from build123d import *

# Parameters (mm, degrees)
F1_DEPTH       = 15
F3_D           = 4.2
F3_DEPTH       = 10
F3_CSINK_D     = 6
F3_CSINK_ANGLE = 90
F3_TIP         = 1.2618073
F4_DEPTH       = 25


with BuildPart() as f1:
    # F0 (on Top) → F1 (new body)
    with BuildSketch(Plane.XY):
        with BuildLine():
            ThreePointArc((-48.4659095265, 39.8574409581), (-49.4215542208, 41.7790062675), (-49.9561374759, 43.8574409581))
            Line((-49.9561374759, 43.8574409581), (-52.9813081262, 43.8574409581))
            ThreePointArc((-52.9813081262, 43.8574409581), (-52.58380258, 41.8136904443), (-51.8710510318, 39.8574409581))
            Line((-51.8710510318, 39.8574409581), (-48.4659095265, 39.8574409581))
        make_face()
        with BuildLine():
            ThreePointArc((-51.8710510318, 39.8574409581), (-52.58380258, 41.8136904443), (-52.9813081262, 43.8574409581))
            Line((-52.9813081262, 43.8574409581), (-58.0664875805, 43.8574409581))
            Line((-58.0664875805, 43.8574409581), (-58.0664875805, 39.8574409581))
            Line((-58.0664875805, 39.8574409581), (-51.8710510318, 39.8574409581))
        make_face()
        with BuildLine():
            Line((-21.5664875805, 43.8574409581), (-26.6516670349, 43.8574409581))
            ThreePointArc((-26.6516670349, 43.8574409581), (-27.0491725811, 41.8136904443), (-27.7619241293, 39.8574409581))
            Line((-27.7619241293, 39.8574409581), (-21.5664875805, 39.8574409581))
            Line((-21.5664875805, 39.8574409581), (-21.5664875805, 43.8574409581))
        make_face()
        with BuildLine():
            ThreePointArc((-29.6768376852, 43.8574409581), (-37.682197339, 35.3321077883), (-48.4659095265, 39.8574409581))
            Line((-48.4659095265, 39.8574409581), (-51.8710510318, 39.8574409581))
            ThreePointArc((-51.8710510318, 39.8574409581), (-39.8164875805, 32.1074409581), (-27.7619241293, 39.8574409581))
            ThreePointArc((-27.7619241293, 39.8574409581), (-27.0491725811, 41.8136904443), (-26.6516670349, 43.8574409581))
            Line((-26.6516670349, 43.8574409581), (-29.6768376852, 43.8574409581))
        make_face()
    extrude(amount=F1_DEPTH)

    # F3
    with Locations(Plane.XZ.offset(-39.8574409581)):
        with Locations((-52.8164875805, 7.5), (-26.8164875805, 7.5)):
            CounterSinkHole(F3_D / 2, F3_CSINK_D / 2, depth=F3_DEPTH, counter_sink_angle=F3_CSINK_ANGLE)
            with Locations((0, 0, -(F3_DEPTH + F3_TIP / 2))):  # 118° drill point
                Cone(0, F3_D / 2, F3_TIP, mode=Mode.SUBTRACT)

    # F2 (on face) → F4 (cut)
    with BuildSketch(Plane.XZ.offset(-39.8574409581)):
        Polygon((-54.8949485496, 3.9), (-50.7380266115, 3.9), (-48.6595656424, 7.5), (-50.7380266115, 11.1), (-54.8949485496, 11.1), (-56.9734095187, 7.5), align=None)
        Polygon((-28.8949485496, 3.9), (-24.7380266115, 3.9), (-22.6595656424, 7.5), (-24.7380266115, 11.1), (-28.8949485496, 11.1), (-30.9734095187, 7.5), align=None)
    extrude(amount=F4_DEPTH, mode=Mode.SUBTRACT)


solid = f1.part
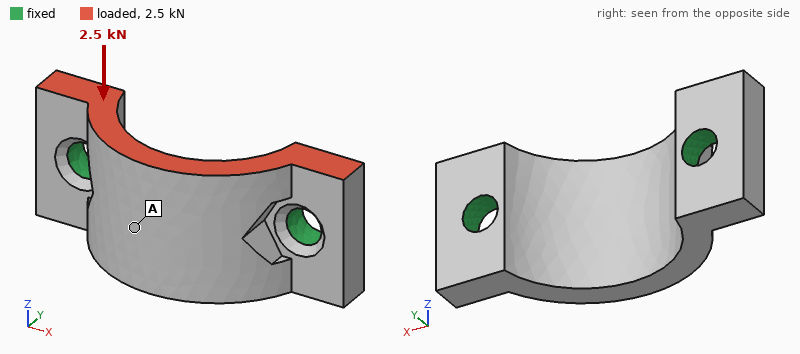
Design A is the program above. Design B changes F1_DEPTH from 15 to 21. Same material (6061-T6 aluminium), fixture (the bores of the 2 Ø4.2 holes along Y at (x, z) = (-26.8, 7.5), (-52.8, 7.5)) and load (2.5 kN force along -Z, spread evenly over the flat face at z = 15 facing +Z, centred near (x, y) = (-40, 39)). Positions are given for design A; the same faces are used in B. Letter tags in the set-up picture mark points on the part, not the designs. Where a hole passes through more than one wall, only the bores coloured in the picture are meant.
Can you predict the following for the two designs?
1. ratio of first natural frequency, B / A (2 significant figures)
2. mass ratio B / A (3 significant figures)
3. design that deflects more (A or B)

0.67
1.44
B
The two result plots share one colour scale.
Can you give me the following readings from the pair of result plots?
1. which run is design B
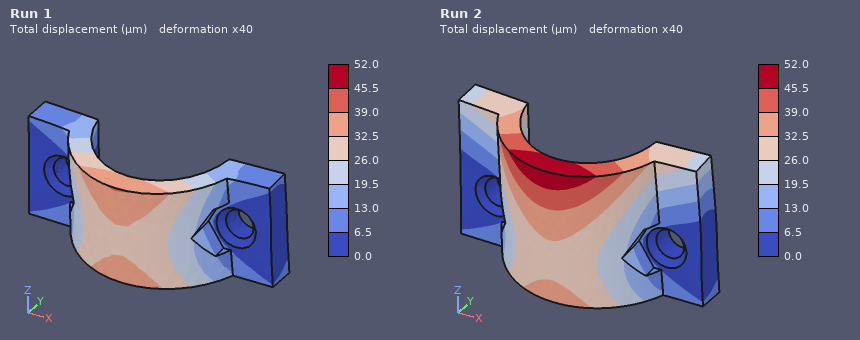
Run 2
